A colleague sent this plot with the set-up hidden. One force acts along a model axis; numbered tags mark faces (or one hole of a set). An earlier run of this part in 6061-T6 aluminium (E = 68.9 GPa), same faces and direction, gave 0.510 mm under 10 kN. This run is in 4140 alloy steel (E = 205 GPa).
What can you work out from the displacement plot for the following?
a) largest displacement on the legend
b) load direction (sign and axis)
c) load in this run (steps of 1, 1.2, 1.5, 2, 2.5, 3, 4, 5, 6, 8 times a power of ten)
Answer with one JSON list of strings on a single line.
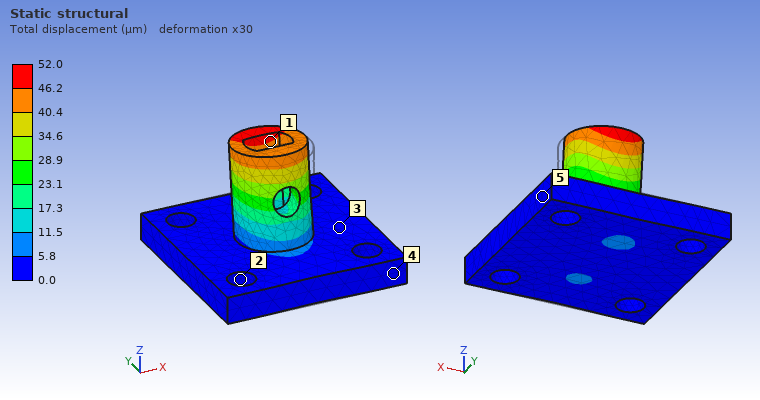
["52.0 µm", "+Y", "3 kN"]
